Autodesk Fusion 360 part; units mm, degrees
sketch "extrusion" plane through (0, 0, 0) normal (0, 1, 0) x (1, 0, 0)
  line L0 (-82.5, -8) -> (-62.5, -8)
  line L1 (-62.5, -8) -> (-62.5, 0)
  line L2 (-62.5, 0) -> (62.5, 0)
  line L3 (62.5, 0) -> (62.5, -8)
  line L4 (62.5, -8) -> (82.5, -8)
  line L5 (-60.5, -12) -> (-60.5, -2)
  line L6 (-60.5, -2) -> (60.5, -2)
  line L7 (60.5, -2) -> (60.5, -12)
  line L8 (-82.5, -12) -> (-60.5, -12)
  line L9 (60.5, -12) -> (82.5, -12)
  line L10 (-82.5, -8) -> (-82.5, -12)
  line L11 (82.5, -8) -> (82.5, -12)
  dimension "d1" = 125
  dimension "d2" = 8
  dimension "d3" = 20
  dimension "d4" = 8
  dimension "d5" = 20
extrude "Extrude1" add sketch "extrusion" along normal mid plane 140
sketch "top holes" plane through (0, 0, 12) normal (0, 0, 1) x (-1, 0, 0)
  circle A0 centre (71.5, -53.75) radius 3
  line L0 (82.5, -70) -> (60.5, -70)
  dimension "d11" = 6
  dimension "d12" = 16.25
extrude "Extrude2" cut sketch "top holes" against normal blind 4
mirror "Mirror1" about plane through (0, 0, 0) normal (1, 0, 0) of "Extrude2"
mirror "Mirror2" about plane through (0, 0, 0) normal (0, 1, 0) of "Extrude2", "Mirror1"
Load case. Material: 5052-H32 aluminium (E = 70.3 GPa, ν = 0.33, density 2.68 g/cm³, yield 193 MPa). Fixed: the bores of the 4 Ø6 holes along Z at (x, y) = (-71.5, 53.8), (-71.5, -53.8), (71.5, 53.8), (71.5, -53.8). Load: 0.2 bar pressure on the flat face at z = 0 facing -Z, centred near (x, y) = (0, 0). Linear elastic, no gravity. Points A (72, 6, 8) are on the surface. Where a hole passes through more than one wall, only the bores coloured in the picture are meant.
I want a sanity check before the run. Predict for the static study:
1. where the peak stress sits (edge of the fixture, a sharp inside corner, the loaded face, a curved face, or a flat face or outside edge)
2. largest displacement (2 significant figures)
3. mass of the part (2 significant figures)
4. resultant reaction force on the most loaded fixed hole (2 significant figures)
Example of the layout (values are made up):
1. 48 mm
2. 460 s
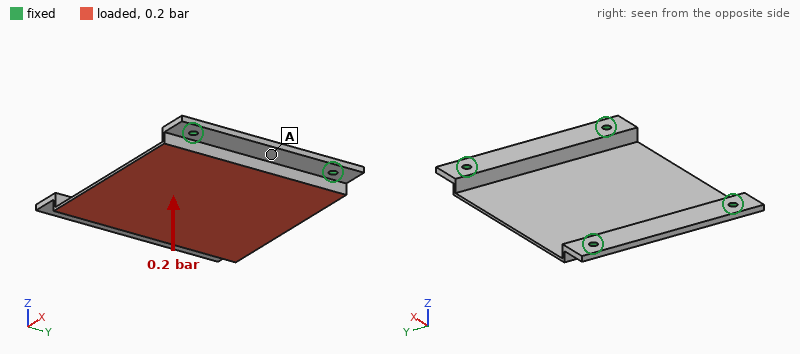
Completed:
1. the loaded face
2. 0.28 mm
3. 170 g
4. 280 N
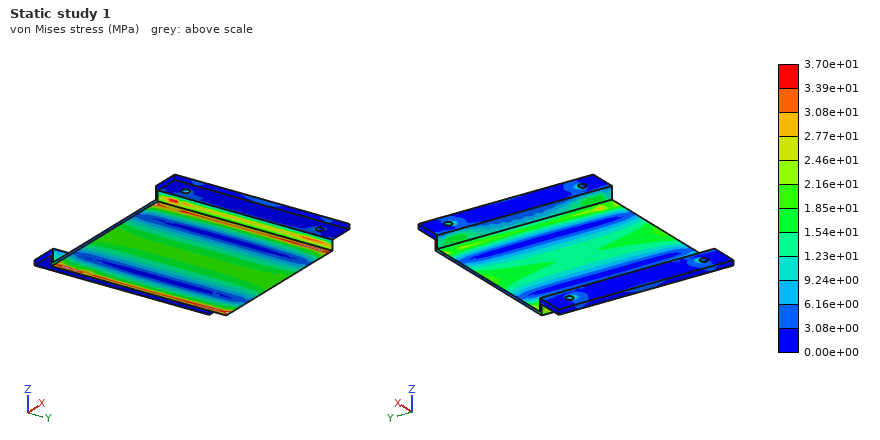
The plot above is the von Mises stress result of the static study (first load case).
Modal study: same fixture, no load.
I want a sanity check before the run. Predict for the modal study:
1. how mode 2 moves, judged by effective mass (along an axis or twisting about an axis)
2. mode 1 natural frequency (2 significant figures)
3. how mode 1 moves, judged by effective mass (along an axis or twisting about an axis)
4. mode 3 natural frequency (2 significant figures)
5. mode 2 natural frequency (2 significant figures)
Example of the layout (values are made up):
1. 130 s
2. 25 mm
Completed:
1. twisting about X
2. 680 Hz
3. along Z
4. 1200 Hz
5. 800 Hz
